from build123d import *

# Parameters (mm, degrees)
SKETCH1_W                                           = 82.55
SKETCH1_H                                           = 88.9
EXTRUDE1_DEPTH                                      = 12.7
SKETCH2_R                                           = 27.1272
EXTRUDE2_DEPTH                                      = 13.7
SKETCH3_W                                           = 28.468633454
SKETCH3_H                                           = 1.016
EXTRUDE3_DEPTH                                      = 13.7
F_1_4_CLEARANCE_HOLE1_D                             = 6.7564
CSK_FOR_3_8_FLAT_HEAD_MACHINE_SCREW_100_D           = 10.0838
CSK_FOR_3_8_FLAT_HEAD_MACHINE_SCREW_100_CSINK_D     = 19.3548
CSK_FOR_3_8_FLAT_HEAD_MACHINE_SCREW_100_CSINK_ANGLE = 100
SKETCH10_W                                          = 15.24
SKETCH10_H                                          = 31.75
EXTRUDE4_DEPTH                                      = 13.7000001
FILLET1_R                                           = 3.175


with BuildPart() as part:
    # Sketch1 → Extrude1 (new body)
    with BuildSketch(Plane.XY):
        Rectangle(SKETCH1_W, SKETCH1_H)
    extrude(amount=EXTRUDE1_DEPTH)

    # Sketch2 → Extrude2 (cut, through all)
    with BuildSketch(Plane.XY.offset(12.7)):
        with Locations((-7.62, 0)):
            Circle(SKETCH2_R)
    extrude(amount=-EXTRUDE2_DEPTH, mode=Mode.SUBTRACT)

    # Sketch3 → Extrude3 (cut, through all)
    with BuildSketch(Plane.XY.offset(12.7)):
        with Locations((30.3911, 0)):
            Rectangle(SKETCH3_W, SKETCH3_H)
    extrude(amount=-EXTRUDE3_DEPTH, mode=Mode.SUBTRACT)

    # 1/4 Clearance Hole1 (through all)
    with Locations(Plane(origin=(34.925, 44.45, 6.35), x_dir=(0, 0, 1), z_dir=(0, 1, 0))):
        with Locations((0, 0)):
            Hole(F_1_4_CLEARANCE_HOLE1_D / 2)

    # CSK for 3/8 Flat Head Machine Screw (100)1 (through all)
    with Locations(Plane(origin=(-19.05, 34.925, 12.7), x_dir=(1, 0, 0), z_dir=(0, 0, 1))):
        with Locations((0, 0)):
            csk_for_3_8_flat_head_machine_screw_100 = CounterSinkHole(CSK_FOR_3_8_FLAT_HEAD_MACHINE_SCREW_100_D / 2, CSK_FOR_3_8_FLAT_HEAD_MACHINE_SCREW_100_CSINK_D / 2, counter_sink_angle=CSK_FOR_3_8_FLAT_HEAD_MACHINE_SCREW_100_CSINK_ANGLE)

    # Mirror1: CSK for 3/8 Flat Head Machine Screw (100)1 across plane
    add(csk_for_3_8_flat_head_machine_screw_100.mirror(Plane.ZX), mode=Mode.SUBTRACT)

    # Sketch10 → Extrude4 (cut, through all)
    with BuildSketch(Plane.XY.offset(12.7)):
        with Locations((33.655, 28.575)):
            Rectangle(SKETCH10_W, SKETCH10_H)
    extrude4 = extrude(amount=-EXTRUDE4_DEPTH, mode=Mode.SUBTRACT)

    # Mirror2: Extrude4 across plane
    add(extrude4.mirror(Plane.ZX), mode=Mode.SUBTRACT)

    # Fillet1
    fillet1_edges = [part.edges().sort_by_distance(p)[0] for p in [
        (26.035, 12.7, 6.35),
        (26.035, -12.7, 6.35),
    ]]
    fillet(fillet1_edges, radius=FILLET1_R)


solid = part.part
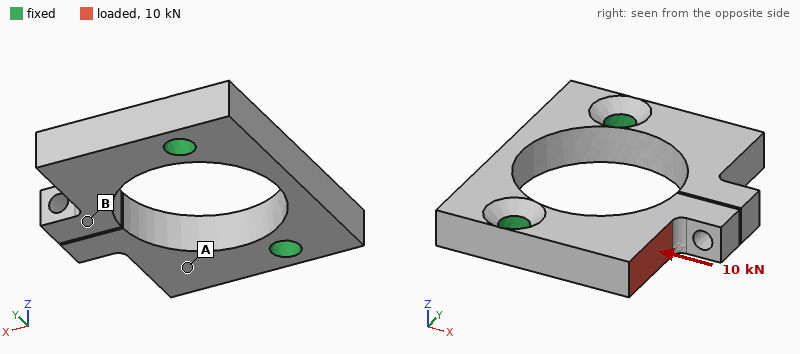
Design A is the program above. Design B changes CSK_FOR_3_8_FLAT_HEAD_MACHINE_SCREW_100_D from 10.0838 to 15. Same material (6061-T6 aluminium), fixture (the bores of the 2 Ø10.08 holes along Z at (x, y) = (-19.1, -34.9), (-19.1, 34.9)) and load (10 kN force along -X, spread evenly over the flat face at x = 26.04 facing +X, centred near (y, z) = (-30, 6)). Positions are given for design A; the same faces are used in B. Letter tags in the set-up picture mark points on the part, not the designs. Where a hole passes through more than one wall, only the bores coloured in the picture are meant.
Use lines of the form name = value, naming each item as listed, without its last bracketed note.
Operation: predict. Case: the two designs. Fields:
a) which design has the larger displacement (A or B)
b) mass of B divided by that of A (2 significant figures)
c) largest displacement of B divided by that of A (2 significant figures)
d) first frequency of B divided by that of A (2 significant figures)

which design has the larger displacement = A
mass of B divided by that of A = 0.96
largest displacement of B divided by that of A = 0.78
first frequency of B divided by that of A = 1.2
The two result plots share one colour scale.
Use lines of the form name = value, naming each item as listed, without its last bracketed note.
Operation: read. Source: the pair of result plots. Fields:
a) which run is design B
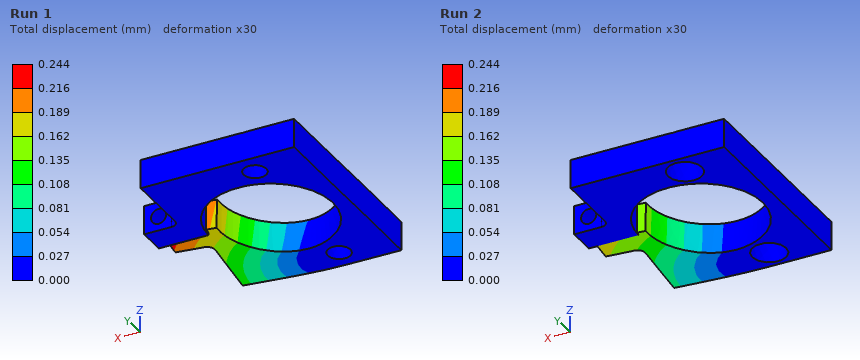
which run is design B = Run 2
